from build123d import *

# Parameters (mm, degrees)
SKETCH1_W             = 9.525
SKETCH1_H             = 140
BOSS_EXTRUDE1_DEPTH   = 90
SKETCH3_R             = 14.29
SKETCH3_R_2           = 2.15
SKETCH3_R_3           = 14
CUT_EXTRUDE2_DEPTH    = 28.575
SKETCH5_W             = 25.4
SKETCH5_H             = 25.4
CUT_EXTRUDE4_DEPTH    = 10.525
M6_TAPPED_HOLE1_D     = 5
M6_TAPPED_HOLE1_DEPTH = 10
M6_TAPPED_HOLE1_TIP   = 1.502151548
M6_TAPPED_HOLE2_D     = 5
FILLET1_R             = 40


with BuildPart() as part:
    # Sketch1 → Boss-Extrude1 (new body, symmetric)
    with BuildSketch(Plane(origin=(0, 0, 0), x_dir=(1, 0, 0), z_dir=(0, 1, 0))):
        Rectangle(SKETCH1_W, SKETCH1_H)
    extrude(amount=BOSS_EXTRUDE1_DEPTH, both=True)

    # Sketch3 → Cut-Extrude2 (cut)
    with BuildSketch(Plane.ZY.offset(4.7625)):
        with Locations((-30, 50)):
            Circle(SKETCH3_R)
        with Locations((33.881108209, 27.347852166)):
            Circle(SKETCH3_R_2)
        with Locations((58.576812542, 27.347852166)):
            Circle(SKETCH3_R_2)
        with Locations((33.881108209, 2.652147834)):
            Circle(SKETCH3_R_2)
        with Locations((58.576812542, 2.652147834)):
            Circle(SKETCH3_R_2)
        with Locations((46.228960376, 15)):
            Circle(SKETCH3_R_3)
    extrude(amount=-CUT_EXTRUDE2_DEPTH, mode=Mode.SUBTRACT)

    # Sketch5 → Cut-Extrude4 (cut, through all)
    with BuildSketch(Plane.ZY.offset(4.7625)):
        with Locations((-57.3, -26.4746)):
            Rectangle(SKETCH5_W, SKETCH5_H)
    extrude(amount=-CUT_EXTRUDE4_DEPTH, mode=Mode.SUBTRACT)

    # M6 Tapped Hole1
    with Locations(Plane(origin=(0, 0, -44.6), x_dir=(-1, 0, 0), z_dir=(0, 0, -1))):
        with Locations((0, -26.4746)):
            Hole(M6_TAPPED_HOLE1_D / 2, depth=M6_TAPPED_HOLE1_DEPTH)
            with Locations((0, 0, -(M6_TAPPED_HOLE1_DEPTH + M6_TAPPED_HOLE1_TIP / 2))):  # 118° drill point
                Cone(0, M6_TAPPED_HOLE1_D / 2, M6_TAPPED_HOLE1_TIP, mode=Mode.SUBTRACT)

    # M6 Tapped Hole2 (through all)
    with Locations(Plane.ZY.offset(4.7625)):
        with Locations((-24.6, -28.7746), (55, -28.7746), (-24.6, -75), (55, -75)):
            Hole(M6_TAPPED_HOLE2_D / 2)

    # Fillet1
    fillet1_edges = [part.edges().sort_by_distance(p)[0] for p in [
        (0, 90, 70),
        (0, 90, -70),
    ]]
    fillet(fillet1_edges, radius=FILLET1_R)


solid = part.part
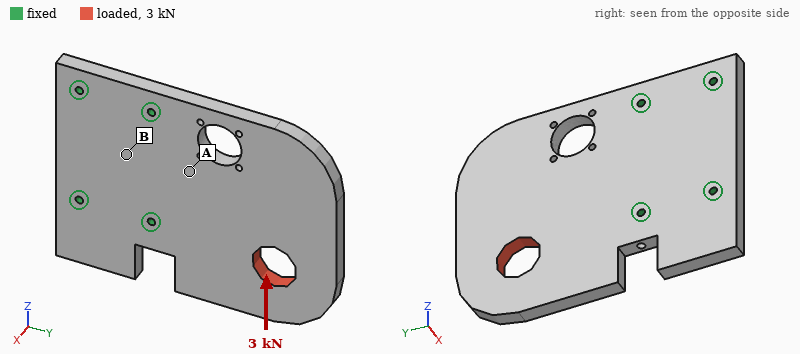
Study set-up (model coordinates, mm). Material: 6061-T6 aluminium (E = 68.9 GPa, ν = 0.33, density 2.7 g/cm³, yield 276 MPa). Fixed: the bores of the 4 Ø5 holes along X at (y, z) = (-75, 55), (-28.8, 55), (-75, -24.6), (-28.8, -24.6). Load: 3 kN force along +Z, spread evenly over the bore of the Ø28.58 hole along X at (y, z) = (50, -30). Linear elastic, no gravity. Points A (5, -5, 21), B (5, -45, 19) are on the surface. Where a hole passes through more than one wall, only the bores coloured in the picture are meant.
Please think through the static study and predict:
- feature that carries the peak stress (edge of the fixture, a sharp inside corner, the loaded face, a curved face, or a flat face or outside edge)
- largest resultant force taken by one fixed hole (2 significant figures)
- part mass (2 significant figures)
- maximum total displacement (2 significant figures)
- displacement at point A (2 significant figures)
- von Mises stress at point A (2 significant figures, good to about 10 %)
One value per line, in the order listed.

a curved face
2.8 kN
580 g
34 µm
5.7 µm
6.4 MPa
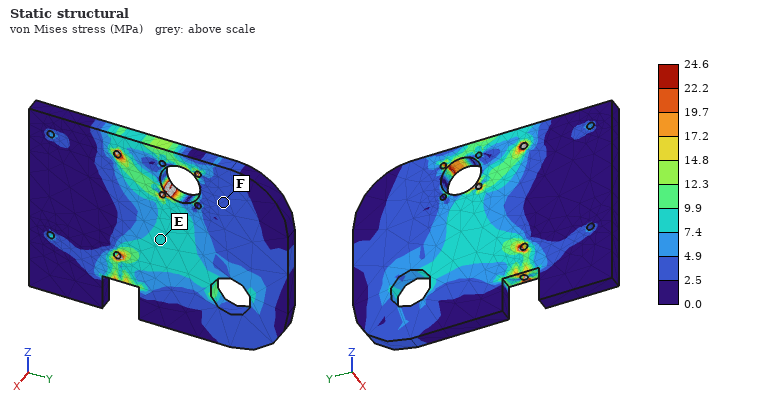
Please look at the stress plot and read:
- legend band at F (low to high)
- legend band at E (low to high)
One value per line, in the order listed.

2.5 to 4.9 MPa
7.4 to 9.9 MPa
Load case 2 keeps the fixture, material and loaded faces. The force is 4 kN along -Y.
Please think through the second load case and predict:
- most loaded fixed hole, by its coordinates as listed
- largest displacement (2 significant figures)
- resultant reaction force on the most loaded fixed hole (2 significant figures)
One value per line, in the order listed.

(-28.8, -24.6)
21 µm
3.2 kN
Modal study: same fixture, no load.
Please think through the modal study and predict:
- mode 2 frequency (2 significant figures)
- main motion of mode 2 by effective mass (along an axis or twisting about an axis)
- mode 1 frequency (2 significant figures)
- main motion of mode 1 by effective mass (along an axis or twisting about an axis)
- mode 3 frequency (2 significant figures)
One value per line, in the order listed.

1100 Hz
twisting about Y
500 Hz
along X
2600 Hz
